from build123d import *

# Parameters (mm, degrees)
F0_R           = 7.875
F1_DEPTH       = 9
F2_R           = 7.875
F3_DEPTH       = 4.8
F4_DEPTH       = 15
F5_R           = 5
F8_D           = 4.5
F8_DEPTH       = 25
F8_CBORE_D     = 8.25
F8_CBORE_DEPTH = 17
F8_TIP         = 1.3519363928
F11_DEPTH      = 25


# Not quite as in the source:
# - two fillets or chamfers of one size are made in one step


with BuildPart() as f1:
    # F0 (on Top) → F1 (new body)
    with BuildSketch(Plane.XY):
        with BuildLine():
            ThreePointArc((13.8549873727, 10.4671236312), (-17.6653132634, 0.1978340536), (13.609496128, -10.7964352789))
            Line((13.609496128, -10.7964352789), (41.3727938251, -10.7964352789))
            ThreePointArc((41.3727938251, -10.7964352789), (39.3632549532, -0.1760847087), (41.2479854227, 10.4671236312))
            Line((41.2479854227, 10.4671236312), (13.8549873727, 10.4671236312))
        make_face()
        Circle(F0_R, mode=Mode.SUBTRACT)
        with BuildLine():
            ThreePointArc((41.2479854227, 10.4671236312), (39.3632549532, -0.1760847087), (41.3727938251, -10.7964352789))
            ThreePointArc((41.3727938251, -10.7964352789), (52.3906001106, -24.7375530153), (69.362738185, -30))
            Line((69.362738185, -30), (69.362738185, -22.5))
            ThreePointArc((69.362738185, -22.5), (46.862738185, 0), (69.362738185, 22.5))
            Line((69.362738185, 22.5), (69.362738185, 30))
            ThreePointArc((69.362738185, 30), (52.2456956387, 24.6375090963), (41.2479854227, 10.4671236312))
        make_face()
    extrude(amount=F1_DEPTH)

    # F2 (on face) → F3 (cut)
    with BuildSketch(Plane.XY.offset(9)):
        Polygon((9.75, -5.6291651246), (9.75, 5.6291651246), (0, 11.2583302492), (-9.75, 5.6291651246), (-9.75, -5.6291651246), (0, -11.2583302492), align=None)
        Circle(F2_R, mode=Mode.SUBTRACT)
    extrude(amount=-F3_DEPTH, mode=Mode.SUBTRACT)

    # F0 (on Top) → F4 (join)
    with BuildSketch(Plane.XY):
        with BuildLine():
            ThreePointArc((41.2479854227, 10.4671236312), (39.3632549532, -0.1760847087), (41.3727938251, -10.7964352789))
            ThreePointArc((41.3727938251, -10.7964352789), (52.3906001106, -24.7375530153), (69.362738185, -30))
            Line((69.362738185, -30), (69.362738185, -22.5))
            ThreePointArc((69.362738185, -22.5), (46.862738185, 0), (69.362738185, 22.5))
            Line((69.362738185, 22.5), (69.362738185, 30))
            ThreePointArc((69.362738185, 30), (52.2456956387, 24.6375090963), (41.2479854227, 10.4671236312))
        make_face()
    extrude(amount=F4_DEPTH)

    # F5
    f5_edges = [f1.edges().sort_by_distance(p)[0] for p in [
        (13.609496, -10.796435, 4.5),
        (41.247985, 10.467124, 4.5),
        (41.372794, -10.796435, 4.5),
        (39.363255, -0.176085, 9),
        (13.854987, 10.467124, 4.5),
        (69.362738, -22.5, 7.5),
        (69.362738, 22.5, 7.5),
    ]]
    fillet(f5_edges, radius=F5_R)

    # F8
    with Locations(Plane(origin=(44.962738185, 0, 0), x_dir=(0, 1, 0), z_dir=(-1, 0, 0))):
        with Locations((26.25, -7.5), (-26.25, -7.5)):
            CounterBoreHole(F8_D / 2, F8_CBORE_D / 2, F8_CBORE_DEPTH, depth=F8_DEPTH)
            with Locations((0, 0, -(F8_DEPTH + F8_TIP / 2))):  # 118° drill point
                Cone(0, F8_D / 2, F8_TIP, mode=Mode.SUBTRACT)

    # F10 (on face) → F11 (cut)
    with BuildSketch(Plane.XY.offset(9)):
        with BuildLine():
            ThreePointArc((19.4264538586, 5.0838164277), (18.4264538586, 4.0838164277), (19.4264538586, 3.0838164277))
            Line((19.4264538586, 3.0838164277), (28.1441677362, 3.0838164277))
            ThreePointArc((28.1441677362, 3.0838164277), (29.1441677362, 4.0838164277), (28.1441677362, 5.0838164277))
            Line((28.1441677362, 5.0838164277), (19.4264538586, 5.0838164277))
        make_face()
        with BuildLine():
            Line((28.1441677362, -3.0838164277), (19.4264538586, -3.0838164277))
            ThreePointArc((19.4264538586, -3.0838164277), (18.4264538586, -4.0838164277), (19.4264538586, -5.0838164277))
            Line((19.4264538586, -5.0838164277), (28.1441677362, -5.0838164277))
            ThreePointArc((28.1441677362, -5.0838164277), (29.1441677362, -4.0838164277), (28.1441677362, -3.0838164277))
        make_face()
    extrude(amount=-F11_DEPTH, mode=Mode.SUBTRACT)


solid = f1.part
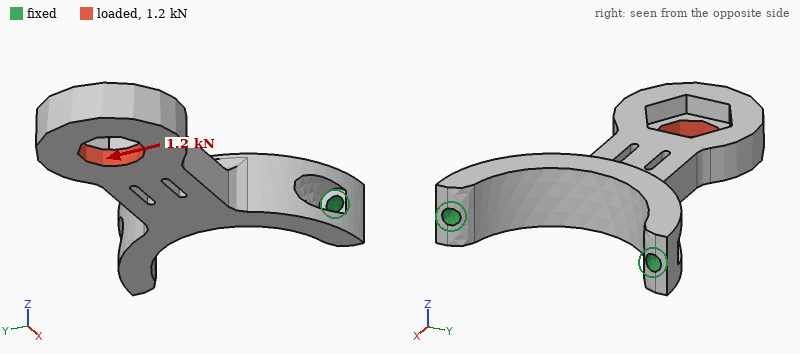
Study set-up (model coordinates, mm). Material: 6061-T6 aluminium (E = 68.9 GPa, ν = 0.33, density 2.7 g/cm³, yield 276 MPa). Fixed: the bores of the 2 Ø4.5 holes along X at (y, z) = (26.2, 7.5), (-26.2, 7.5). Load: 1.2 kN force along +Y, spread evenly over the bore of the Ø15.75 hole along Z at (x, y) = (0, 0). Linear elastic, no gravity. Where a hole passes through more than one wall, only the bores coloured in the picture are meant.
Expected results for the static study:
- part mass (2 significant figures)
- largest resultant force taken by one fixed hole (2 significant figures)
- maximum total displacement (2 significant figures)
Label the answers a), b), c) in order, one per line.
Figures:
a) 51 g
b) 1.7 kN
c) 0.24 mm
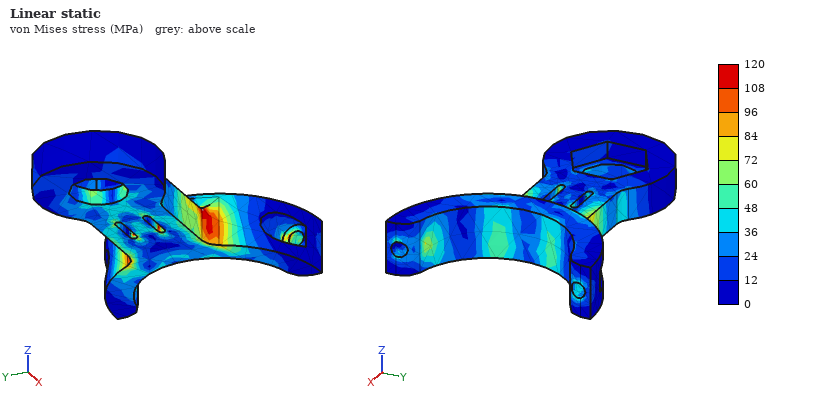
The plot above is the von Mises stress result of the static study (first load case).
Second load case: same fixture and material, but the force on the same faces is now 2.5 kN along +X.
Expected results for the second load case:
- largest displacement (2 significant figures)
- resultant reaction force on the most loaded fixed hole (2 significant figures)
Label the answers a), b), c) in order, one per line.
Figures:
a) 0.32 mm
b) 1.5 kN
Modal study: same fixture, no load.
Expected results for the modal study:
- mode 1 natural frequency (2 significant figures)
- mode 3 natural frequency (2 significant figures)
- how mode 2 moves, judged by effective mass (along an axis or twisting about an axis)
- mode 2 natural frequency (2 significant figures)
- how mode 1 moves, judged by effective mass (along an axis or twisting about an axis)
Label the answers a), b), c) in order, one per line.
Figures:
a) 1200 Hz
b) 4900 Hz
c) along Y
d) 3000 Hz
e) along Z
